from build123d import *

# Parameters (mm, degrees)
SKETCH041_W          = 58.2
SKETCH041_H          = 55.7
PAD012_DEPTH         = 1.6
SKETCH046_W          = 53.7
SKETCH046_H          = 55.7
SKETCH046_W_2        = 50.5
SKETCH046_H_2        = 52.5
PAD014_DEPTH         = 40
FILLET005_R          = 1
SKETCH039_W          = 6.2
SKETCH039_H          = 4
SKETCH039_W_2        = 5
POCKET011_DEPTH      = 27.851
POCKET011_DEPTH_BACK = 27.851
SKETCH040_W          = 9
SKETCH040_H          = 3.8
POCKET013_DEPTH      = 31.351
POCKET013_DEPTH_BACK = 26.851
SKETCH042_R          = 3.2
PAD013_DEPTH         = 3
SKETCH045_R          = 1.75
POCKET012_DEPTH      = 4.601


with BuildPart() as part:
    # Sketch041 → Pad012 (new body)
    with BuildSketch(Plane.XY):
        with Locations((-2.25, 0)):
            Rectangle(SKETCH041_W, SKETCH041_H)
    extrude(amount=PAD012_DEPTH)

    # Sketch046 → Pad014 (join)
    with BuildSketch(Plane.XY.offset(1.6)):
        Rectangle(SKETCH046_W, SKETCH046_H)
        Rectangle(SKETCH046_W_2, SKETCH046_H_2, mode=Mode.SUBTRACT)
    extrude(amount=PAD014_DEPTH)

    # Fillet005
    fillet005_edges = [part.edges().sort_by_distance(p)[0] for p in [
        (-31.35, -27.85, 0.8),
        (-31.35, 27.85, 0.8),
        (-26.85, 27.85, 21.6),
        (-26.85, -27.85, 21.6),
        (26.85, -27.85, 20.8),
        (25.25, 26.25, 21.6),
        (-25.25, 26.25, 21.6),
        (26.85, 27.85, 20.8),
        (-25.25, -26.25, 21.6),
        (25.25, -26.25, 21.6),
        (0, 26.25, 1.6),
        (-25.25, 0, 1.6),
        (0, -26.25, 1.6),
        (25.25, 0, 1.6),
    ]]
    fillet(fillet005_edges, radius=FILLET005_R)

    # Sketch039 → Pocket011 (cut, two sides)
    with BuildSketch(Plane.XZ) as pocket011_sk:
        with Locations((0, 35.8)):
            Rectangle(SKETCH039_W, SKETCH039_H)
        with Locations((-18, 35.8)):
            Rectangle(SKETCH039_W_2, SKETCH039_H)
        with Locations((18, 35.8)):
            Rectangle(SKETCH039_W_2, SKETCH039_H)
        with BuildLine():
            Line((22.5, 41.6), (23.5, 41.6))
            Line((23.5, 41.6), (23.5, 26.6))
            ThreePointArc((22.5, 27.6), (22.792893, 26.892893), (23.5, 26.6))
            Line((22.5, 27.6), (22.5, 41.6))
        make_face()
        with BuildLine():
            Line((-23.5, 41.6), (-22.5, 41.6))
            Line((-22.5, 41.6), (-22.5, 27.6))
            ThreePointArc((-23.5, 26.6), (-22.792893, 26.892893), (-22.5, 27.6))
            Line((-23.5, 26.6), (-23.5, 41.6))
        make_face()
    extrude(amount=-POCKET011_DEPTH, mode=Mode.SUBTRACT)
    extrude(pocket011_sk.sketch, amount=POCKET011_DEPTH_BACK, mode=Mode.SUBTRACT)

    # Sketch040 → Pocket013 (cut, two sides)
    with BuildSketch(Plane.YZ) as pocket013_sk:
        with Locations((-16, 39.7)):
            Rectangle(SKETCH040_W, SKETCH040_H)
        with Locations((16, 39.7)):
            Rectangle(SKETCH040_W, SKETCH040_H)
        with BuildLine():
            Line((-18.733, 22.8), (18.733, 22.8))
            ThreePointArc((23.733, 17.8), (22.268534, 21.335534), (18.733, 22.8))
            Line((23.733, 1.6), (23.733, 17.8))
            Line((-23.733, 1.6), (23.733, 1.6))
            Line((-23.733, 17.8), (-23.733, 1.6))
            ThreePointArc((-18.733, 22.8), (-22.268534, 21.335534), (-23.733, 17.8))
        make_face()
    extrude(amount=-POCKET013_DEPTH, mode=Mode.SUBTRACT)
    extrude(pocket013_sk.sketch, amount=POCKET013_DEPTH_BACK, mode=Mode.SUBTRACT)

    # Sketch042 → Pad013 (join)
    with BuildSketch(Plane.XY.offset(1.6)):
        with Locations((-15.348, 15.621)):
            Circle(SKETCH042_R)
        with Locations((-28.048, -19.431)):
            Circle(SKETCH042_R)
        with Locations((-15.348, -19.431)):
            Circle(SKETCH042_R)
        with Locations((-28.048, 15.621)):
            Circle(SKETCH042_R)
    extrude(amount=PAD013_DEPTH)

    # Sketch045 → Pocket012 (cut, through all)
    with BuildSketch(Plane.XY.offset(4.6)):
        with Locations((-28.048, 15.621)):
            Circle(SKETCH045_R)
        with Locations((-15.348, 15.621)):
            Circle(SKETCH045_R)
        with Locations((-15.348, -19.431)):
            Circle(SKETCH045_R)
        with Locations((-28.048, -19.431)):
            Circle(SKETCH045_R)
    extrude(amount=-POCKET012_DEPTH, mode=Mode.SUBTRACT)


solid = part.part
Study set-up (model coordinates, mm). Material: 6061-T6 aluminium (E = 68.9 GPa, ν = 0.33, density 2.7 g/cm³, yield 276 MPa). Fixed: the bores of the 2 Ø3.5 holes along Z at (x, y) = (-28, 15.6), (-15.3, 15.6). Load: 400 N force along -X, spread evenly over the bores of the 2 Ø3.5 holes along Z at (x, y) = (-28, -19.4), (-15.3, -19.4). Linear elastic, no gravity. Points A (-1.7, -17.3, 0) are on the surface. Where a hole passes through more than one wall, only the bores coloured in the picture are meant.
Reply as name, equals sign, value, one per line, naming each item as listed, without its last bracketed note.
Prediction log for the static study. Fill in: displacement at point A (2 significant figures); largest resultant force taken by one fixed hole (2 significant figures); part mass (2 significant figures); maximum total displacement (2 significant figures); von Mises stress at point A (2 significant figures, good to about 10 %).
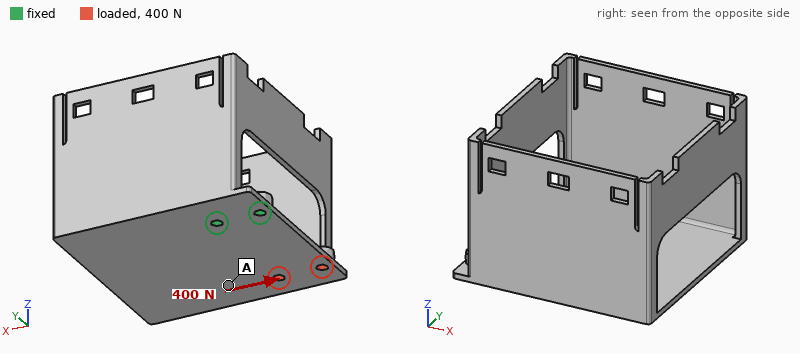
displacement at point A = 0.068 mm
largest resultant force taken by one fixed hole = 920 N
part mass = 41 g
maximum total displacement = 0.26 mm
von Mises stress at point A = 4.9 MPa
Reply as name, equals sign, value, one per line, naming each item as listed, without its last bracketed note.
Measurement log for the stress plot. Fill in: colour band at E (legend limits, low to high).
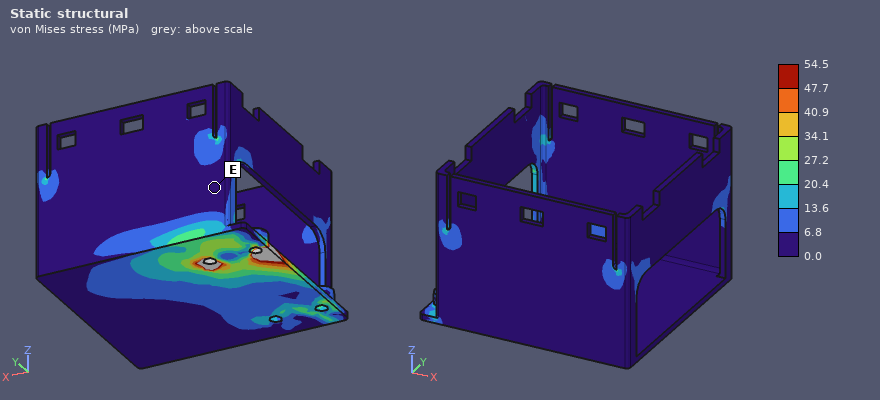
colour band at E = 0.0 to 6.8 MPa
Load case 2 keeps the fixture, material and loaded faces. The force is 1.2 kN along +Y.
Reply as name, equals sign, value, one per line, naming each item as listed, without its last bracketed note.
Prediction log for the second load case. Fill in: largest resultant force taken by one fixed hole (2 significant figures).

largest resultant force taken by one fixed hole = 610 N
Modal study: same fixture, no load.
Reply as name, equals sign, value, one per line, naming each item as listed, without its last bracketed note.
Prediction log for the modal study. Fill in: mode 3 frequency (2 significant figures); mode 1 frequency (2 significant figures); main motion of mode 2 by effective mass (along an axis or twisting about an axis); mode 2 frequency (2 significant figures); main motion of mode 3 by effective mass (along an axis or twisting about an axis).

mode 3 frequency = 810 Hz
mode 1 frequency = 280 Hz
main motion of mode 2 by effective mass = along X
mode 2 frequency = 480 Hz
main motion of mode 3 by effective mass = along Z
